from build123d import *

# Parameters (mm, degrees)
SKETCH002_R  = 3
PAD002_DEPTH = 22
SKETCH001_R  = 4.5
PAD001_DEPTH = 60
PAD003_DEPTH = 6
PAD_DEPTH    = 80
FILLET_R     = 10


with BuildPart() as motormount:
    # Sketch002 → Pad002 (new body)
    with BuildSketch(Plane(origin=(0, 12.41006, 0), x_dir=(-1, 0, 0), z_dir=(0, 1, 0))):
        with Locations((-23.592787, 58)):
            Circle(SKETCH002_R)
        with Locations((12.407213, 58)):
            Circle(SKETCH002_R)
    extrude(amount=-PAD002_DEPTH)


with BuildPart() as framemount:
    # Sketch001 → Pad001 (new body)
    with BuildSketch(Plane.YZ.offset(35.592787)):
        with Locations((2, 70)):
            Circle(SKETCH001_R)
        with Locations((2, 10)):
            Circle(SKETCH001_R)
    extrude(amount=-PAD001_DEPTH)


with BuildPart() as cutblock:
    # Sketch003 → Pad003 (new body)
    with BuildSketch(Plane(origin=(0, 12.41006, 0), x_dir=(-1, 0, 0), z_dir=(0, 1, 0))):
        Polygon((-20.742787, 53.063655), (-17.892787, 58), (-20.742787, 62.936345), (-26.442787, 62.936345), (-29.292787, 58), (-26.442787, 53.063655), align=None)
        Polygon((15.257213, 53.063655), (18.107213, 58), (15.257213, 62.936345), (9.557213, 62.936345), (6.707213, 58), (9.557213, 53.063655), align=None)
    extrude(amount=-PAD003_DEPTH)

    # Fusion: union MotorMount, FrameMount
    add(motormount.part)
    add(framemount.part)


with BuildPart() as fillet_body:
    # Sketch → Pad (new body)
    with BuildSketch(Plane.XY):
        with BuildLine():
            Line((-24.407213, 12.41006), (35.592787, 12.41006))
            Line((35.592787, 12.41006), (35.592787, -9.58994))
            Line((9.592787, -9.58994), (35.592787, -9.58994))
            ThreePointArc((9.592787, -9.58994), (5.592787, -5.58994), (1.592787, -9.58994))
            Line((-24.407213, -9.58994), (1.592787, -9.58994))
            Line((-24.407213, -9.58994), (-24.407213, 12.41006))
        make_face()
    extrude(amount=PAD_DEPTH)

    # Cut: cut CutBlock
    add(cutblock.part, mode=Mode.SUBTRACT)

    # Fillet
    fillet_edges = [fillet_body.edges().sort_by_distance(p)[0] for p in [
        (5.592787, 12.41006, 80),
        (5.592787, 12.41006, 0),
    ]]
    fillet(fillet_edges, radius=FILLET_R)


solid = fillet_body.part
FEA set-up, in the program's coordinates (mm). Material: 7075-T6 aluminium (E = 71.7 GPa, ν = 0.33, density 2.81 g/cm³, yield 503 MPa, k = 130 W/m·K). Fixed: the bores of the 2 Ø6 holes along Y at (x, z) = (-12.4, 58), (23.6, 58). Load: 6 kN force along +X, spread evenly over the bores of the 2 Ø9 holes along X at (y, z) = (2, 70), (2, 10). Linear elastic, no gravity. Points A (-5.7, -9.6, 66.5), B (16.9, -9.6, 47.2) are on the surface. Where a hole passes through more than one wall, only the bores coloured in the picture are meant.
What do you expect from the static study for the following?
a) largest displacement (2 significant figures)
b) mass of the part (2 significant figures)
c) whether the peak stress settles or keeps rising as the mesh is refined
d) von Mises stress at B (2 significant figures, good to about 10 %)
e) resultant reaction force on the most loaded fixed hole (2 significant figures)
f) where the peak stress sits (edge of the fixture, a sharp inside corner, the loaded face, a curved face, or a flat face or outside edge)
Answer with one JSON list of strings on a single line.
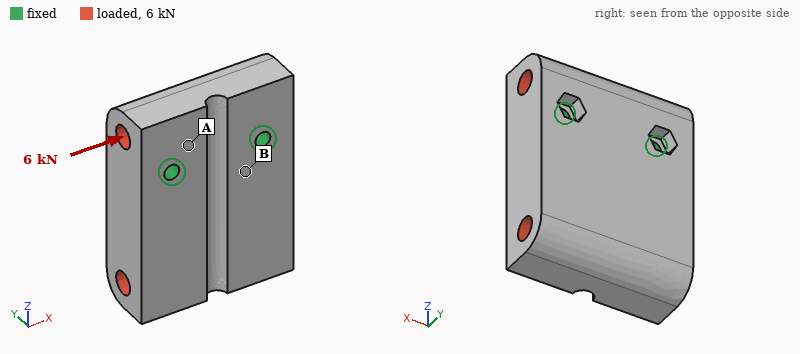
["14 µm", "260 g", "keeps rising", "7.9 MPa", "4.1 kN", "edge of the fixture"]
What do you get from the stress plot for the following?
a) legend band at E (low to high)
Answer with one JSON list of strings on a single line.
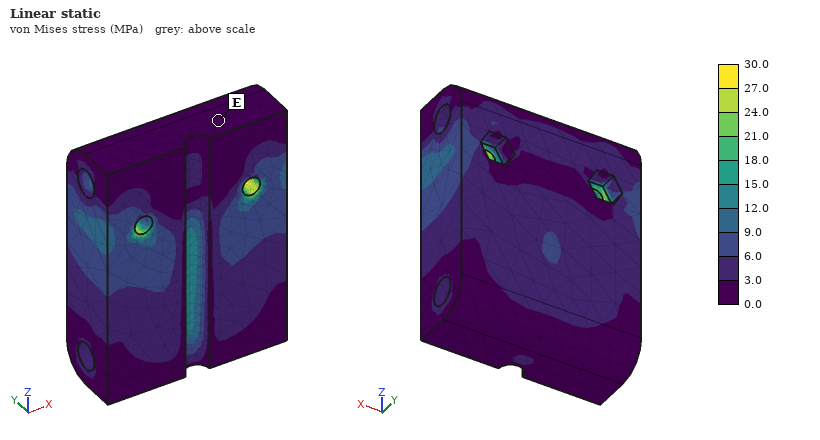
["0.0 to 3.0 MPa"]
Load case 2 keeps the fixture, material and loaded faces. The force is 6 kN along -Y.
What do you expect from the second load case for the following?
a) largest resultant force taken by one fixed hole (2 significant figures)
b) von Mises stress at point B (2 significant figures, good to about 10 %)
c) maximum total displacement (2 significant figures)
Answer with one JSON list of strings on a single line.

["3.0 kN", "26 MPa", "72 µm"]
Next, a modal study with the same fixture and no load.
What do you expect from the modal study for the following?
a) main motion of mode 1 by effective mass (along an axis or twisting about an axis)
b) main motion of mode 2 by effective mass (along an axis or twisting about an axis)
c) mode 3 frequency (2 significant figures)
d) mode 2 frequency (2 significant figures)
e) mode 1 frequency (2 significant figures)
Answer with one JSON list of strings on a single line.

["along Y", "along X", "9100 Hz", "8000 Hz", "3800 Hz"]
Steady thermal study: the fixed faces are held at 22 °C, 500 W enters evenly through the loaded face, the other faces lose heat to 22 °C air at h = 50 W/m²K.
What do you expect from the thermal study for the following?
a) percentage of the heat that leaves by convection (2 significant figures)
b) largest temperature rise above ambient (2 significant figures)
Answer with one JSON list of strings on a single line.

["7.0 %", "86 K"]
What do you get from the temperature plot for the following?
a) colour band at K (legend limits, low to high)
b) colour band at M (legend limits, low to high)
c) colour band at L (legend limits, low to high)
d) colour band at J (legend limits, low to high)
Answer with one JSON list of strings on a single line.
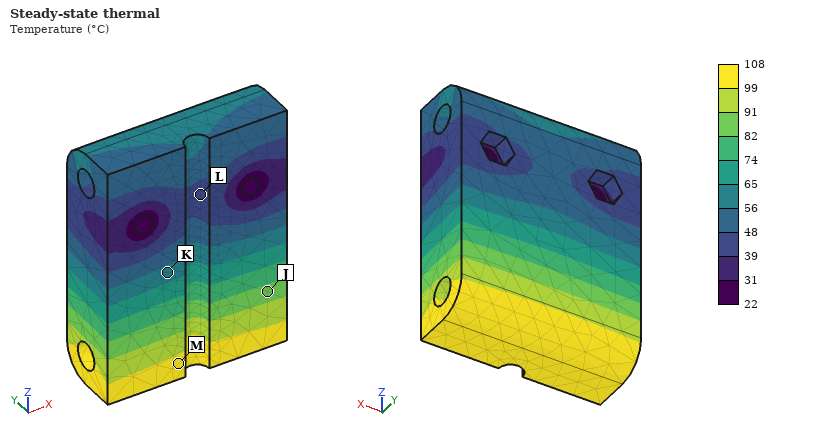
["56 to 65 °C", "99 to 108 °C", "39 to 48 °C", "82 to 91 °C"]
